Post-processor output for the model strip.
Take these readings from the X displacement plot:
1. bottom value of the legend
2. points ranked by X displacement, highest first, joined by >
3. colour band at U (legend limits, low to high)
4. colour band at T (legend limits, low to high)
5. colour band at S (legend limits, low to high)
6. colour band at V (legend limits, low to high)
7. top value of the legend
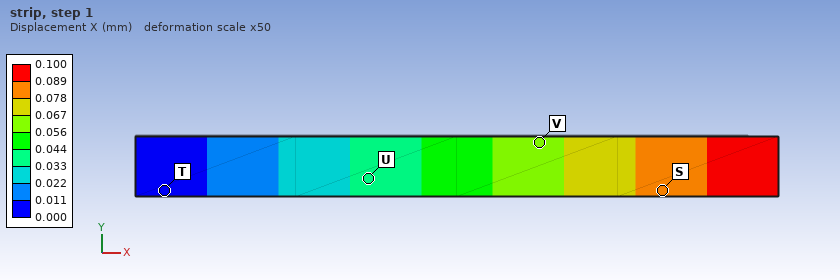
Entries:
0.000 mm
S > V > U > T
0.033 to 0.044 mm
0.000 to 0.011 mm
0.078 to 0.089 mm
0.056 to 0.067 mm
0.100 mm
